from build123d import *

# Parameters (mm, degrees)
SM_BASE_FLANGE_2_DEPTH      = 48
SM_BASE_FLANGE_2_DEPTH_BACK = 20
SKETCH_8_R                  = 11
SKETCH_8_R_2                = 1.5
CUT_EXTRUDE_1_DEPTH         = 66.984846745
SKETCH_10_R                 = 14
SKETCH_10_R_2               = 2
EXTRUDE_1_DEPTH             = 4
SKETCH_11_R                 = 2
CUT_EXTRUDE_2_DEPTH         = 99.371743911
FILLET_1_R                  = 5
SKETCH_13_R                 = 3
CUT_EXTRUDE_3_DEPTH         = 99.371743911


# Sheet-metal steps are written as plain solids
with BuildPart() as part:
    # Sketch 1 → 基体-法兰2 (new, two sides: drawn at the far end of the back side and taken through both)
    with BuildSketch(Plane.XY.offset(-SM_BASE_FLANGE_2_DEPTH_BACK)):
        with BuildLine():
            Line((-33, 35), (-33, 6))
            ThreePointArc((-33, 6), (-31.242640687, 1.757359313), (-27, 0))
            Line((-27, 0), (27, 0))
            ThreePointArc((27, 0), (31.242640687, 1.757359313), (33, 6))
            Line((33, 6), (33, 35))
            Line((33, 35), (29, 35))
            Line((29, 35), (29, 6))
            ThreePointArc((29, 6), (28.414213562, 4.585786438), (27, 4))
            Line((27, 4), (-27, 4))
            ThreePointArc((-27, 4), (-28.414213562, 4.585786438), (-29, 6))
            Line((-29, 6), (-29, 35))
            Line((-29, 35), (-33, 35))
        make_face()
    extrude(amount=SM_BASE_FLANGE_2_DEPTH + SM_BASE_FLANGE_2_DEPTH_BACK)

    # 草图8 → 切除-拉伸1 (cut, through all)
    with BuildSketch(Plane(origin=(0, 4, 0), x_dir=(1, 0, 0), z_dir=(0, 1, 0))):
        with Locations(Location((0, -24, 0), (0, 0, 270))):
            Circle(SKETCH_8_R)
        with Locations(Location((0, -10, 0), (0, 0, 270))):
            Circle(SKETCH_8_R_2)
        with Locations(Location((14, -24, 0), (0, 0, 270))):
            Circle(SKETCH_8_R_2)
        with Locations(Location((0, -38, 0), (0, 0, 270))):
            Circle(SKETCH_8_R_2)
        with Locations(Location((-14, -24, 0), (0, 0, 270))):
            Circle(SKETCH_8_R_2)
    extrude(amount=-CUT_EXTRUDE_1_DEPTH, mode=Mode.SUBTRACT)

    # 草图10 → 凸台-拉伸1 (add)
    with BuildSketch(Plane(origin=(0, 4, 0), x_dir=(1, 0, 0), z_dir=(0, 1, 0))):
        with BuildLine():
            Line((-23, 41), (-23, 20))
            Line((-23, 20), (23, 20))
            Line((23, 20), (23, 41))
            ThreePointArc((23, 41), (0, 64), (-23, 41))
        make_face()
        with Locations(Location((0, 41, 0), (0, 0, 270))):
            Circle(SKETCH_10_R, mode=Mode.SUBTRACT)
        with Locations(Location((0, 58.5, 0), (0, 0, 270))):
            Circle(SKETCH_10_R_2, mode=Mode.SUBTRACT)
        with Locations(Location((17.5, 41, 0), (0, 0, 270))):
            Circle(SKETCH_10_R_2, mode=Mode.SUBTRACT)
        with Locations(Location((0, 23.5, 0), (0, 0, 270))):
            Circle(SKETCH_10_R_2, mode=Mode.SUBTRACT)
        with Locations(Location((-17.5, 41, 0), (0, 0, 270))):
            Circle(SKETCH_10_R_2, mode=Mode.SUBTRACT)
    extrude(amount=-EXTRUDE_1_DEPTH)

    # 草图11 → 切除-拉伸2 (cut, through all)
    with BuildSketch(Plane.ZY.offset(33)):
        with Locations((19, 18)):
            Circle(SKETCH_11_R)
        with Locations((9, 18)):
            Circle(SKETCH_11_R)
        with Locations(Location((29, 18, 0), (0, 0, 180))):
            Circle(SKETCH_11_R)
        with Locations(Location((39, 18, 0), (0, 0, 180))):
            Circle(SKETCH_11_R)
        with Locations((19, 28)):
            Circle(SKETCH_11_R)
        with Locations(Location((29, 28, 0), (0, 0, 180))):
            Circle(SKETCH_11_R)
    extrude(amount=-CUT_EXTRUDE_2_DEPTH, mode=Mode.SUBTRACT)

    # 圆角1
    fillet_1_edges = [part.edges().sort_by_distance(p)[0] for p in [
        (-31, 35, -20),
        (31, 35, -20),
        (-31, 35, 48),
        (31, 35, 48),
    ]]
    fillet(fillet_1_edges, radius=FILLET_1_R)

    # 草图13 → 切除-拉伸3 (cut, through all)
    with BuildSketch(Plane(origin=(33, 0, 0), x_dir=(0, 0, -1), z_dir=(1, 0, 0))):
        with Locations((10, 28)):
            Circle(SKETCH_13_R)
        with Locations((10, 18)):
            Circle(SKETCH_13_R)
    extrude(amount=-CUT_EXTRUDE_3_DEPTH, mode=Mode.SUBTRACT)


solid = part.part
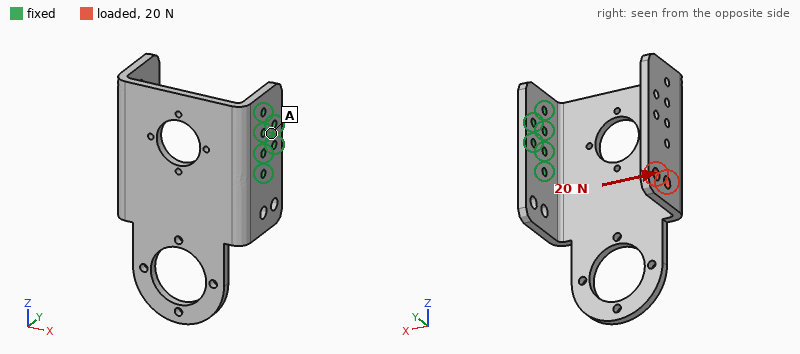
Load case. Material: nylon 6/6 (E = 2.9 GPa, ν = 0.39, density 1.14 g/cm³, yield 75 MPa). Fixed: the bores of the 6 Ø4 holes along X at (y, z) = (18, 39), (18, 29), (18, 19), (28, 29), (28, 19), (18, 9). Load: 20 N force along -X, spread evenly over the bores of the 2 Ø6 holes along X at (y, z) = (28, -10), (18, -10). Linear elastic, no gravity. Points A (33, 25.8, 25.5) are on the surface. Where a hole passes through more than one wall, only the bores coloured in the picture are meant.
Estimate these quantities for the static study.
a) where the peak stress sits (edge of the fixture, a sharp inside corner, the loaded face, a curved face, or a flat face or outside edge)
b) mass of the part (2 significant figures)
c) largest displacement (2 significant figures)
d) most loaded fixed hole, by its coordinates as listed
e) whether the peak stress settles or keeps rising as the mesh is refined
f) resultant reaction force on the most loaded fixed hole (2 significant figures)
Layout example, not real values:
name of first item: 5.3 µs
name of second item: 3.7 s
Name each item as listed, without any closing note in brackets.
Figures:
where the peak stress sits: a sharp inside corner
mass of the part: 41 g
largest displacement: 1.6 mm
most loaded fixed hole, by its coordinates as listed: (18, 9)
whether the peak stress settles or keeps rising as the mesh is refined: keeps rising
resultant reaction force on the most loaded fixed hole: 29 N
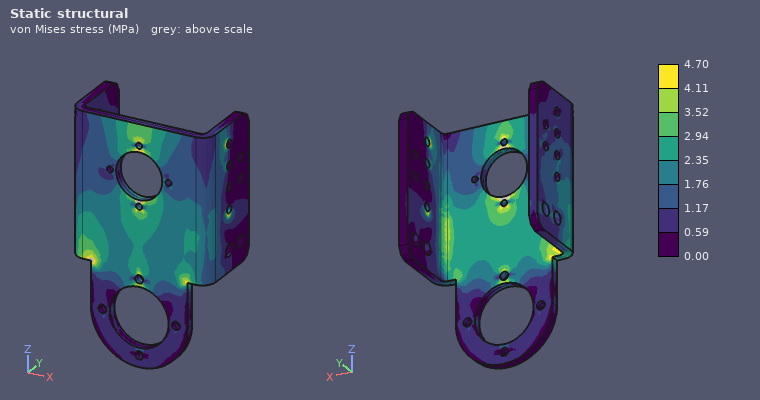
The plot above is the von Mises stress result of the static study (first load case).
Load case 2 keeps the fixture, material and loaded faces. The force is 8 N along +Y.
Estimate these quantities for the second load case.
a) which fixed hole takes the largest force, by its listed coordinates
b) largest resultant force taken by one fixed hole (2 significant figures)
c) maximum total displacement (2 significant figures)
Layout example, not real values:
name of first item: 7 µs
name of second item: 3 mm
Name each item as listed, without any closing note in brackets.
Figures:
which fixed hole takes the largest force, by its listed coordinates: (18, 9)
largest resultant force taken by one fixed hole: 10 N
maximum total displacement: 1.5 mm
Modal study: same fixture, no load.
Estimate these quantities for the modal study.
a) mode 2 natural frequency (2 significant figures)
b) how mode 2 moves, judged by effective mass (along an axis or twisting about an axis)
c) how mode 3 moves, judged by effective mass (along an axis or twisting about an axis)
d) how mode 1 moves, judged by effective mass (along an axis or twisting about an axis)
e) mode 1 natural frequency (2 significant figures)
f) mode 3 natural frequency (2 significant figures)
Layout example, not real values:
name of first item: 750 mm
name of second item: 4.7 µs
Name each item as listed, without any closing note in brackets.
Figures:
mode 2 natural frequency: 200 Hz
how mode 2 moves, judged by effective mass: along Z
how mode 3 moves, judged by effective mass: along Z
how mode 1 moves, judged by effective mass: along Y
mode 1 natural frequency: 110 Hz
mode 3 natural frequency: 340 Hz
